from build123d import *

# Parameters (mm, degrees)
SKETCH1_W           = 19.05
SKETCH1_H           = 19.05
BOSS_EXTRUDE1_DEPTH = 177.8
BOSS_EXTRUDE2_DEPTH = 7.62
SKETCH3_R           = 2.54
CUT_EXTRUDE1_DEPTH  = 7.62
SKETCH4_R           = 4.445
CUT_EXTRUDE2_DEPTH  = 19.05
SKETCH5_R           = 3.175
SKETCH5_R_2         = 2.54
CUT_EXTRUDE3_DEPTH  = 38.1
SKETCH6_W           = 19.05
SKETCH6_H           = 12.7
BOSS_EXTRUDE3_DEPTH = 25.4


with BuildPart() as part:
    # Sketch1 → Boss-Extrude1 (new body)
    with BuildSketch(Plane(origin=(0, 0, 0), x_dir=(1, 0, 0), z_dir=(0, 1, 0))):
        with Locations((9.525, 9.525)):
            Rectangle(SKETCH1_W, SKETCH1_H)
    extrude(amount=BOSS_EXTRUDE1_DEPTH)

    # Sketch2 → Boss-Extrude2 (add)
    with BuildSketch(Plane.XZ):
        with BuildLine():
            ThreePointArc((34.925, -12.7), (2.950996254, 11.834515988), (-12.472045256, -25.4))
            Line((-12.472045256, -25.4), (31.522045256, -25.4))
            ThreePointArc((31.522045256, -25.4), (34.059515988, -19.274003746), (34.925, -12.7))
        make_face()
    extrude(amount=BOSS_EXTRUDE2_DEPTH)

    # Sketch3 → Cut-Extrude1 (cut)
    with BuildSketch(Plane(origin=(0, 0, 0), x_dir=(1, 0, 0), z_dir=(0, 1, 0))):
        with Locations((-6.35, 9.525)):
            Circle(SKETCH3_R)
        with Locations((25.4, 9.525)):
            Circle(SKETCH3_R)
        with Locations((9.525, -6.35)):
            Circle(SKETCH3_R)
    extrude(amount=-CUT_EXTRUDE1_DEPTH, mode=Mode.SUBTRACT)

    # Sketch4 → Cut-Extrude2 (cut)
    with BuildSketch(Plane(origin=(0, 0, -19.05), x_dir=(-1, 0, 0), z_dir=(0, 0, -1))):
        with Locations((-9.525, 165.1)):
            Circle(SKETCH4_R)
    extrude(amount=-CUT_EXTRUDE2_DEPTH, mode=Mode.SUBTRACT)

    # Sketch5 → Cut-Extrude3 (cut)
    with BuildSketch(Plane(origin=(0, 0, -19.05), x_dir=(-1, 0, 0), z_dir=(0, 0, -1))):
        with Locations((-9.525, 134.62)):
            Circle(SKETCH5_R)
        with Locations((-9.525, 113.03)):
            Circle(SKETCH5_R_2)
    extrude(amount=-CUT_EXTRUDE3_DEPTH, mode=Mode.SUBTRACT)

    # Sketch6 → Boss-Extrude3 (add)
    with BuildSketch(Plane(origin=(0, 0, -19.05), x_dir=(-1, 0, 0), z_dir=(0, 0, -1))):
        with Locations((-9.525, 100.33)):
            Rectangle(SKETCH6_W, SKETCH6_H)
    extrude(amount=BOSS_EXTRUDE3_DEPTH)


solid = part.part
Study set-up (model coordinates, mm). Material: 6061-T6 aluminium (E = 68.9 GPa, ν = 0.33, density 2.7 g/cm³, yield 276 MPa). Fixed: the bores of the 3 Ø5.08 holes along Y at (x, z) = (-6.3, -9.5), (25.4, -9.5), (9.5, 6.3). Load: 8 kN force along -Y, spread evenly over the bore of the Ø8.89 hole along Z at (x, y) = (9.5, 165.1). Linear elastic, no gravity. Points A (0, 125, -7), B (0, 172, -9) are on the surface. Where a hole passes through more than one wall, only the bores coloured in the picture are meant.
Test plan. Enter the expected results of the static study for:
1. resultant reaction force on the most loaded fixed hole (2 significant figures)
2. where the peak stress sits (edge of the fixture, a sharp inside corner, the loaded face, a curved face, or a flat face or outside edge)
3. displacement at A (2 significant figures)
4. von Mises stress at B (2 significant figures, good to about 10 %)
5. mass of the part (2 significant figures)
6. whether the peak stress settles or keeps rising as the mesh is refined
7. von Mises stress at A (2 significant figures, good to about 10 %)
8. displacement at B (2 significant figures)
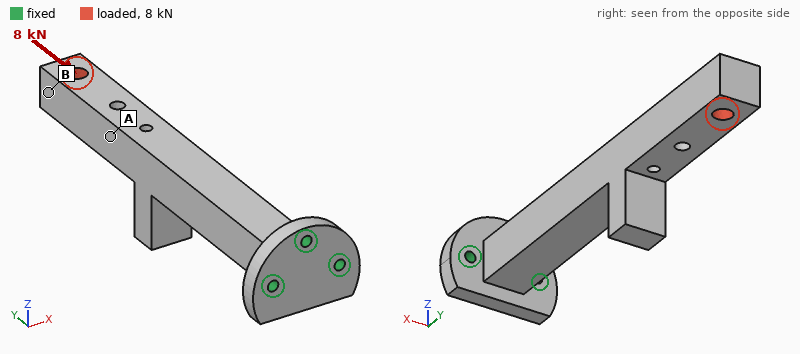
3.3 kN
edge of the fixture
0.11 mm
8.4 MPa
220 g
keeps rising
29 MPa
0.14 mm
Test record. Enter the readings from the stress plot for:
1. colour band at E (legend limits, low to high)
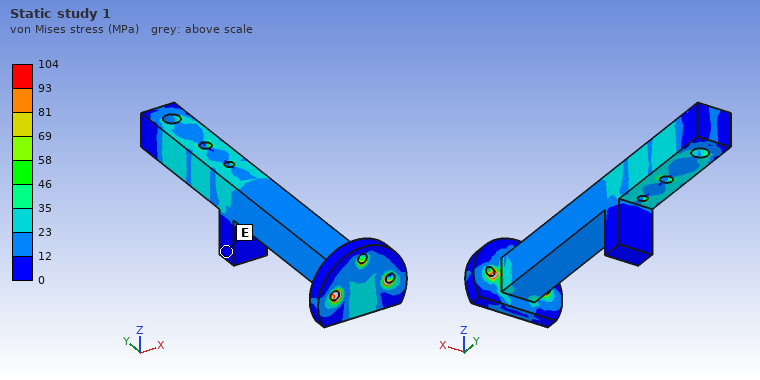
0 to 12 MPa
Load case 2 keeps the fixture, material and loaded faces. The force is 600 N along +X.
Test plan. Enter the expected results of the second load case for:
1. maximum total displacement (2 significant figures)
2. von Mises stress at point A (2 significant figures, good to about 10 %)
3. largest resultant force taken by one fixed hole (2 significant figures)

1.5 mm
22 MPa
3.5 kN
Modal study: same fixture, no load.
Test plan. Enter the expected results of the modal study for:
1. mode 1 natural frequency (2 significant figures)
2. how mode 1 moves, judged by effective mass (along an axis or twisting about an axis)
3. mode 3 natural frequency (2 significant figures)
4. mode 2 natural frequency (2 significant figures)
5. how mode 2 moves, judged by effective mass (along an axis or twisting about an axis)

410 Hz
along Z
2400 Hz
450 Hz
along X
